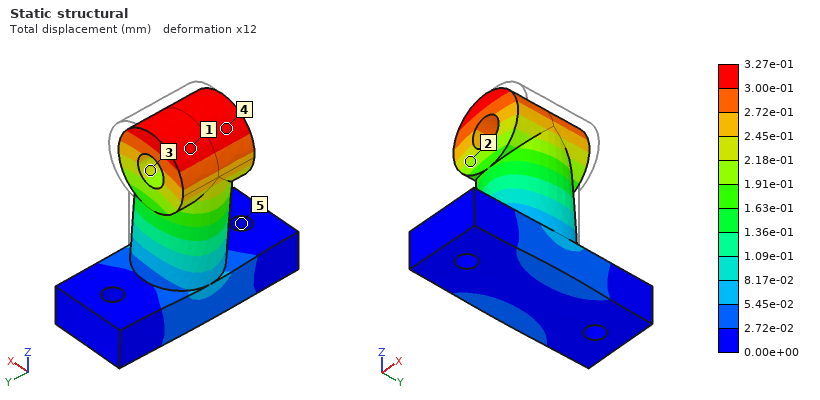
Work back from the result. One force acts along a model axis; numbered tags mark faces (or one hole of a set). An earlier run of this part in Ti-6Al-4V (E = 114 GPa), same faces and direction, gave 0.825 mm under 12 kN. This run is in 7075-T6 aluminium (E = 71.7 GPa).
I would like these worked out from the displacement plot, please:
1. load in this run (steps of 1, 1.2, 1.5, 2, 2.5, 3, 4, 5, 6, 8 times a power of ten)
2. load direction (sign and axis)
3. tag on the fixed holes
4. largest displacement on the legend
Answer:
3 kN
-X
5
3.27e-01 mm
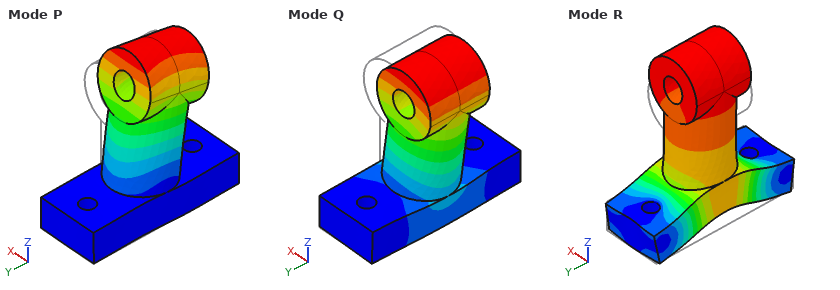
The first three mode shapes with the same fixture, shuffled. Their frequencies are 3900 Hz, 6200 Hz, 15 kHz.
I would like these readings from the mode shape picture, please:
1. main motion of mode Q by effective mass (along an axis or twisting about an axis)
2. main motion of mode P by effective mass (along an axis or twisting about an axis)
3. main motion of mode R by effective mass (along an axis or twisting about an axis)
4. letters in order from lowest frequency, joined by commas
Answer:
along X
along Y
along Z
Q, P, R
